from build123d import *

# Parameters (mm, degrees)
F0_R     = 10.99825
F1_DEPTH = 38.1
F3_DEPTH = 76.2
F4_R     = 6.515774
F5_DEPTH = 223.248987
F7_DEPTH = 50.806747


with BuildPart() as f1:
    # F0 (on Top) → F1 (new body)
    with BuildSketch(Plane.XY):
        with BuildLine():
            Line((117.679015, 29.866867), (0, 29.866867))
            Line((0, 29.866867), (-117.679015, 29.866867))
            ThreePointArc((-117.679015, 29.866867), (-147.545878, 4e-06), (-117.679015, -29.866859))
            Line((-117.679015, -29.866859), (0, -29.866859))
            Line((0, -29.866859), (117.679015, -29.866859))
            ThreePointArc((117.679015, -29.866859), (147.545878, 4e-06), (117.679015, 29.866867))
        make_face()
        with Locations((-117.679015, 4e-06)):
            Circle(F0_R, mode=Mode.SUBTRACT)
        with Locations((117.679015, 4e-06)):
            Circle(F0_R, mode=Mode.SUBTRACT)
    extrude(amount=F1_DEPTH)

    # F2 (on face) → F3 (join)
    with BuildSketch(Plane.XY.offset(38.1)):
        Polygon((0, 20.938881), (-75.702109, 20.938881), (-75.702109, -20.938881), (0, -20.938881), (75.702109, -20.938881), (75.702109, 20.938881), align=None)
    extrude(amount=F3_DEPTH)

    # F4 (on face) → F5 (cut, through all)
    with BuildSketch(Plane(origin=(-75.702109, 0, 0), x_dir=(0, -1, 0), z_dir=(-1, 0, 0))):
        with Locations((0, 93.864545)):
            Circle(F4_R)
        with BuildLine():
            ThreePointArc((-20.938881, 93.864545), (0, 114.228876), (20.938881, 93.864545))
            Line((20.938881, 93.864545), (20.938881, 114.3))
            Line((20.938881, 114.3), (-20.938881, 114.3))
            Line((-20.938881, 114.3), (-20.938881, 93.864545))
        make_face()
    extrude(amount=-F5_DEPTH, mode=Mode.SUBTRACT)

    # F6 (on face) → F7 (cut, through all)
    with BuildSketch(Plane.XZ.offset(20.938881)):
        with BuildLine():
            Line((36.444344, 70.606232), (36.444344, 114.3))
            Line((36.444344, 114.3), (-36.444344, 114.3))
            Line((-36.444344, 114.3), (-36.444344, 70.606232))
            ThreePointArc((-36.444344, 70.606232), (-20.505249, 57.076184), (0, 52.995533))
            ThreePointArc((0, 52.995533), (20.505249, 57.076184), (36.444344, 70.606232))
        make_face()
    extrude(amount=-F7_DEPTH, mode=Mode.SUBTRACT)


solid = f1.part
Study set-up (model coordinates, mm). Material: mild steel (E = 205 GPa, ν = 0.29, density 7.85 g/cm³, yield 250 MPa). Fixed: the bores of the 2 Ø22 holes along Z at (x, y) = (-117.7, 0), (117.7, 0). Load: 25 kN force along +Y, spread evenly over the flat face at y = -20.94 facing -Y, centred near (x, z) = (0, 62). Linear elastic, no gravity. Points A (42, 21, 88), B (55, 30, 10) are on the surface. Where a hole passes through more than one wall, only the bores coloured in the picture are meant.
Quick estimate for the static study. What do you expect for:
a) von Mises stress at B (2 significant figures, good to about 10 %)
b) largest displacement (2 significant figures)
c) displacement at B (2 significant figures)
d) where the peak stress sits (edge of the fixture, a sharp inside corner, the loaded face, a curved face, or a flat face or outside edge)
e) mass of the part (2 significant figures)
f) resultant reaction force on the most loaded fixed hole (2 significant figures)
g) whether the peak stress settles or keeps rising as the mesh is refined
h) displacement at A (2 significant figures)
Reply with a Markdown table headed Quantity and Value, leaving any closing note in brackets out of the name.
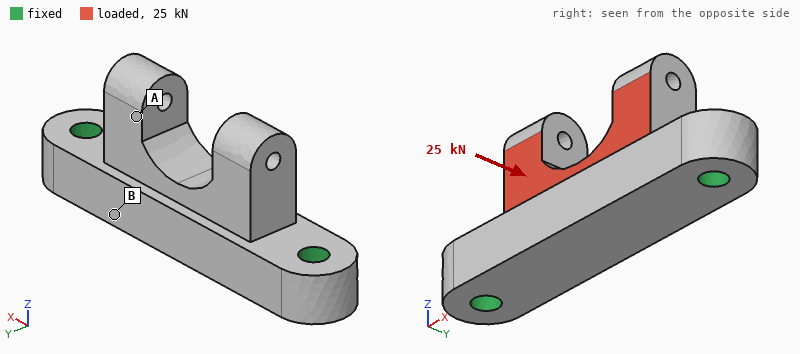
| Quantity | Value |
|---|---|
| von Mises stress at B | 16 MPa |
| largest displacement | 68 µm |
| displacement at B | 15 µm |
| where the peak stress sits | edge of the fixture |
| mass of the part | 7.1 kg |
| resultant reaction force on the most loaded fixed hole | 13 kN |
| whether the peak stress settles or keeps rising as the mesh is refined | keeps rising |
| displacement at A | 53 µm |
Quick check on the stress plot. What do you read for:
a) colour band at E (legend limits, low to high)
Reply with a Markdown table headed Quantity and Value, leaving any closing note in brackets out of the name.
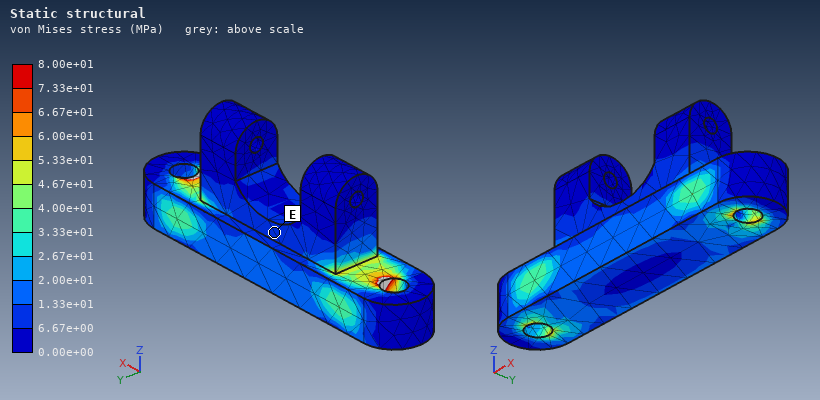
| Quantity | Value |
|---|---|
| colour band at E | 6.67e+00 to 1.33e+01 MPa |
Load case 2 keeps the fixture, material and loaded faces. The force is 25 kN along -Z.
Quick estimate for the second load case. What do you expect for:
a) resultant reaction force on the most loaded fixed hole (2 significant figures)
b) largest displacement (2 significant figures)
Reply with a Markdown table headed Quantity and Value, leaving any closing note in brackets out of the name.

| Quantity | Value |
|---|---|
| resultant reaction force on the most loaded fixed hole | 13 kN |
| largest displacement | 35 µm |
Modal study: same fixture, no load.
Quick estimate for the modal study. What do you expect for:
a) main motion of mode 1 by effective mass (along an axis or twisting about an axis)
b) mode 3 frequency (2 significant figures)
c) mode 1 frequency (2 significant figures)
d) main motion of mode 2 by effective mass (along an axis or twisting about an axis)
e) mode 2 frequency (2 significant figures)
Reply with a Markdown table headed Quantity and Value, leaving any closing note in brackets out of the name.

| Quantity | Value |
|---|---|
| main motion of mode 1 by effective mass | along Y |
| mode 3 frequency | 3800 Hz |
| mode 1 frequency | 2200 Hz |
| main motion of mode 2 by effective mass | along Z |
| mode 2 frequency | 3000 Hz |
